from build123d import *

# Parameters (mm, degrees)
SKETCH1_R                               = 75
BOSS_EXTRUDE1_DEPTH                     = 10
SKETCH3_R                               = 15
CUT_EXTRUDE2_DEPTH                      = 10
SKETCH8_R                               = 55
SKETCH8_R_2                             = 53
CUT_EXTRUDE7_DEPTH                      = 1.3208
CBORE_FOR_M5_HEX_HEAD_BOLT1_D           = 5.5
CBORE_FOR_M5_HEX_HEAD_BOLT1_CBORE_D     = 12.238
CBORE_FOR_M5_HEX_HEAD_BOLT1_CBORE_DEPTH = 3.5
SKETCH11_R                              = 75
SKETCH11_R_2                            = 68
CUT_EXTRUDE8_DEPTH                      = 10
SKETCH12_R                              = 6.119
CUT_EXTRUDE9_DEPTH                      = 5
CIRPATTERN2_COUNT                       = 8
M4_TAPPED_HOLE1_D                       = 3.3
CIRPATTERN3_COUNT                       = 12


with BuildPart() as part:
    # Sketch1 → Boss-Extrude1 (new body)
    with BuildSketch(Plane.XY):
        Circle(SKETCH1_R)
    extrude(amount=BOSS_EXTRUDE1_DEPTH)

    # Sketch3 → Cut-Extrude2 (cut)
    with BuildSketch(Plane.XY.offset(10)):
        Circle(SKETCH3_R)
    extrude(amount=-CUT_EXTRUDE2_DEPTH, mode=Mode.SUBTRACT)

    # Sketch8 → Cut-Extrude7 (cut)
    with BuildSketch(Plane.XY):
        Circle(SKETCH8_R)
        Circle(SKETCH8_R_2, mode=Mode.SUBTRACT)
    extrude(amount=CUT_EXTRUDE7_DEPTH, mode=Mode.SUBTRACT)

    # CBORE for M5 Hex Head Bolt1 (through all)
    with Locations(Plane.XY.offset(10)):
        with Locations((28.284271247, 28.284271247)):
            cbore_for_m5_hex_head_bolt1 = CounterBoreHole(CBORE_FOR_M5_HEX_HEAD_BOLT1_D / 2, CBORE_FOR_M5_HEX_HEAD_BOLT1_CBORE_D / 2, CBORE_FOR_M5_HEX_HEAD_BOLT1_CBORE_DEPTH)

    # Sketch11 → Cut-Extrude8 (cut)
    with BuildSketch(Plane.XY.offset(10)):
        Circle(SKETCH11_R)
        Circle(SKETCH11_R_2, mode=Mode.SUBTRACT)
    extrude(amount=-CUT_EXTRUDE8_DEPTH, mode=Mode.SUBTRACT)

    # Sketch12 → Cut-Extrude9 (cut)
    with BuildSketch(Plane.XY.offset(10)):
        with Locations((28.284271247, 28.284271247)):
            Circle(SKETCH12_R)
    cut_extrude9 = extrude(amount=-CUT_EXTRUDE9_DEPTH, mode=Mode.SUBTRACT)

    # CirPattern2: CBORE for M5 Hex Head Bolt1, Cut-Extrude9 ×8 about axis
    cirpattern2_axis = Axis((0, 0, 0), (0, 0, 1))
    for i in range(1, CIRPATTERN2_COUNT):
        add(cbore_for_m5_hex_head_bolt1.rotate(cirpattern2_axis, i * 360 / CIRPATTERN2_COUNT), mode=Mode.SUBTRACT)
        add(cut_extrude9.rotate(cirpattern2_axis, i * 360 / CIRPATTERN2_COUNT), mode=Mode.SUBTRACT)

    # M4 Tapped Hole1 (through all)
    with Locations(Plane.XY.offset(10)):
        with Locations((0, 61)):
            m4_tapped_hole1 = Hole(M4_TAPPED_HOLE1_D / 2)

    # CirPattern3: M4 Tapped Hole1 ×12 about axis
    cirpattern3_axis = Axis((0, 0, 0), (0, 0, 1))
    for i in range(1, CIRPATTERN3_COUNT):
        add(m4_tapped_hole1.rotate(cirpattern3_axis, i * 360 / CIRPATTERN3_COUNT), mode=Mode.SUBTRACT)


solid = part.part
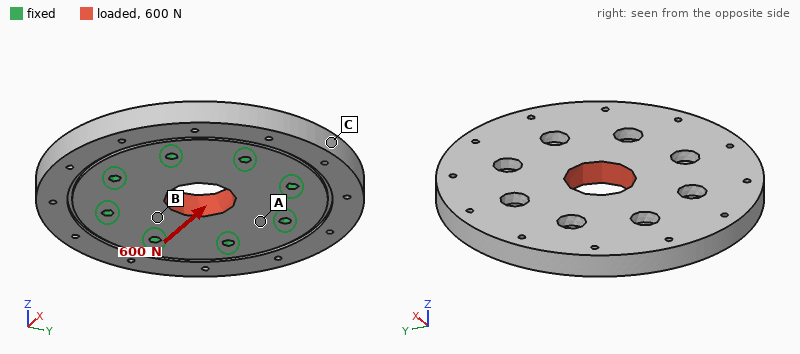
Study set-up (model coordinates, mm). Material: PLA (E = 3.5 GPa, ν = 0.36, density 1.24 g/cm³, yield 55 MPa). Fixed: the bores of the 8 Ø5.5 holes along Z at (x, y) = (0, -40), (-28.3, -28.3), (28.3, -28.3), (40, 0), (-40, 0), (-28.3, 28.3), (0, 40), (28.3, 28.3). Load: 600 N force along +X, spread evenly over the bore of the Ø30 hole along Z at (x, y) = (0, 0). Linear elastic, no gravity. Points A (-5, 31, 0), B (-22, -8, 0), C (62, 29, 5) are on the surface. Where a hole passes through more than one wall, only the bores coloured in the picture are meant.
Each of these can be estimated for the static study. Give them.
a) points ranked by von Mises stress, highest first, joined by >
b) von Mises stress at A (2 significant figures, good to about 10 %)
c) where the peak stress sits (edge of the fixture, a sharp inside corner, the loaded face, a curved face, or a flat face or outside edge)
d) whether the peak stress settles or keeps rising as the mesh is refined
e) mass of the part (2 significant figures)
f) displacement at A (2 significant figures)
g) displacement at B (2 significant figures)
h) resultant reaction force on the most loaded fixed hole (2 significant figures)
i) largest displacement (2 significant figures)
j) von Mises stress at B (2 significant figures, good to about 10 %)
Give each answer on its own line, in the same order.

B > A > C
0.36 MPa
edge of the fixture
keeps rising
160 g
1.7 µm
4.2 µm
110 N
7.3 µm
0.62 MPa
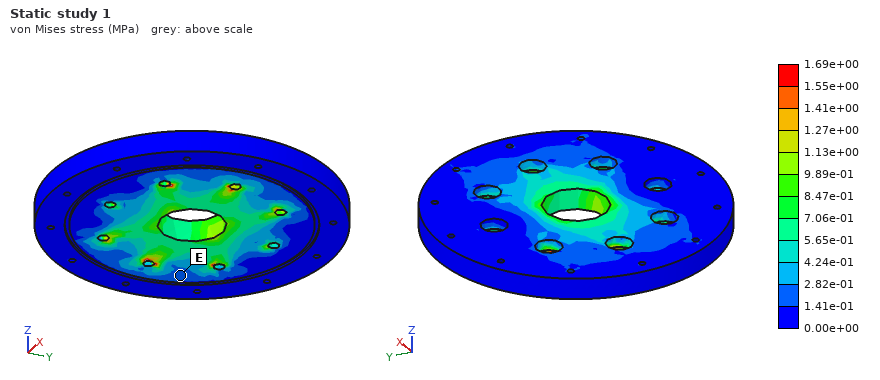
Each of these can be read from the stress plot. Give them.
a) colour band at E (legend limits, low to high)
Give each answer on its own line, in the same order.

1.41e-01 to 2.82e-01 MPa
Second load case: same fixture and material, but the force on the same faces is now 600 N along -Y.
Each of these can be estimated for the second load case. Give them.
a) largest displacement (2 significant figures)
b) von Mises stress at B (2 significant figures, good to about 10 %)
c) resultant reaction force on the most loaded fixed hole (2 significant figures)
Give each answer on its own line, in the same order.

7.2 µm
0.60 MPa
110 N
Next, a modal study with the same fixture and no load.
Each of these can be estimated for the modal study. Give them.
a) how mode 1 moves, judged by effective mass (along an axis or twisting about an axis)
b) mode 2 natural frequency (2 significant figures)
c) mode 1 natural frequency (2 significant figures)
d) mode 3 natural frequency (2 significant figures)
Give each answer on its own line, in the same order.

along Z
2000 Hz
1900 Hz
2000 Hz
